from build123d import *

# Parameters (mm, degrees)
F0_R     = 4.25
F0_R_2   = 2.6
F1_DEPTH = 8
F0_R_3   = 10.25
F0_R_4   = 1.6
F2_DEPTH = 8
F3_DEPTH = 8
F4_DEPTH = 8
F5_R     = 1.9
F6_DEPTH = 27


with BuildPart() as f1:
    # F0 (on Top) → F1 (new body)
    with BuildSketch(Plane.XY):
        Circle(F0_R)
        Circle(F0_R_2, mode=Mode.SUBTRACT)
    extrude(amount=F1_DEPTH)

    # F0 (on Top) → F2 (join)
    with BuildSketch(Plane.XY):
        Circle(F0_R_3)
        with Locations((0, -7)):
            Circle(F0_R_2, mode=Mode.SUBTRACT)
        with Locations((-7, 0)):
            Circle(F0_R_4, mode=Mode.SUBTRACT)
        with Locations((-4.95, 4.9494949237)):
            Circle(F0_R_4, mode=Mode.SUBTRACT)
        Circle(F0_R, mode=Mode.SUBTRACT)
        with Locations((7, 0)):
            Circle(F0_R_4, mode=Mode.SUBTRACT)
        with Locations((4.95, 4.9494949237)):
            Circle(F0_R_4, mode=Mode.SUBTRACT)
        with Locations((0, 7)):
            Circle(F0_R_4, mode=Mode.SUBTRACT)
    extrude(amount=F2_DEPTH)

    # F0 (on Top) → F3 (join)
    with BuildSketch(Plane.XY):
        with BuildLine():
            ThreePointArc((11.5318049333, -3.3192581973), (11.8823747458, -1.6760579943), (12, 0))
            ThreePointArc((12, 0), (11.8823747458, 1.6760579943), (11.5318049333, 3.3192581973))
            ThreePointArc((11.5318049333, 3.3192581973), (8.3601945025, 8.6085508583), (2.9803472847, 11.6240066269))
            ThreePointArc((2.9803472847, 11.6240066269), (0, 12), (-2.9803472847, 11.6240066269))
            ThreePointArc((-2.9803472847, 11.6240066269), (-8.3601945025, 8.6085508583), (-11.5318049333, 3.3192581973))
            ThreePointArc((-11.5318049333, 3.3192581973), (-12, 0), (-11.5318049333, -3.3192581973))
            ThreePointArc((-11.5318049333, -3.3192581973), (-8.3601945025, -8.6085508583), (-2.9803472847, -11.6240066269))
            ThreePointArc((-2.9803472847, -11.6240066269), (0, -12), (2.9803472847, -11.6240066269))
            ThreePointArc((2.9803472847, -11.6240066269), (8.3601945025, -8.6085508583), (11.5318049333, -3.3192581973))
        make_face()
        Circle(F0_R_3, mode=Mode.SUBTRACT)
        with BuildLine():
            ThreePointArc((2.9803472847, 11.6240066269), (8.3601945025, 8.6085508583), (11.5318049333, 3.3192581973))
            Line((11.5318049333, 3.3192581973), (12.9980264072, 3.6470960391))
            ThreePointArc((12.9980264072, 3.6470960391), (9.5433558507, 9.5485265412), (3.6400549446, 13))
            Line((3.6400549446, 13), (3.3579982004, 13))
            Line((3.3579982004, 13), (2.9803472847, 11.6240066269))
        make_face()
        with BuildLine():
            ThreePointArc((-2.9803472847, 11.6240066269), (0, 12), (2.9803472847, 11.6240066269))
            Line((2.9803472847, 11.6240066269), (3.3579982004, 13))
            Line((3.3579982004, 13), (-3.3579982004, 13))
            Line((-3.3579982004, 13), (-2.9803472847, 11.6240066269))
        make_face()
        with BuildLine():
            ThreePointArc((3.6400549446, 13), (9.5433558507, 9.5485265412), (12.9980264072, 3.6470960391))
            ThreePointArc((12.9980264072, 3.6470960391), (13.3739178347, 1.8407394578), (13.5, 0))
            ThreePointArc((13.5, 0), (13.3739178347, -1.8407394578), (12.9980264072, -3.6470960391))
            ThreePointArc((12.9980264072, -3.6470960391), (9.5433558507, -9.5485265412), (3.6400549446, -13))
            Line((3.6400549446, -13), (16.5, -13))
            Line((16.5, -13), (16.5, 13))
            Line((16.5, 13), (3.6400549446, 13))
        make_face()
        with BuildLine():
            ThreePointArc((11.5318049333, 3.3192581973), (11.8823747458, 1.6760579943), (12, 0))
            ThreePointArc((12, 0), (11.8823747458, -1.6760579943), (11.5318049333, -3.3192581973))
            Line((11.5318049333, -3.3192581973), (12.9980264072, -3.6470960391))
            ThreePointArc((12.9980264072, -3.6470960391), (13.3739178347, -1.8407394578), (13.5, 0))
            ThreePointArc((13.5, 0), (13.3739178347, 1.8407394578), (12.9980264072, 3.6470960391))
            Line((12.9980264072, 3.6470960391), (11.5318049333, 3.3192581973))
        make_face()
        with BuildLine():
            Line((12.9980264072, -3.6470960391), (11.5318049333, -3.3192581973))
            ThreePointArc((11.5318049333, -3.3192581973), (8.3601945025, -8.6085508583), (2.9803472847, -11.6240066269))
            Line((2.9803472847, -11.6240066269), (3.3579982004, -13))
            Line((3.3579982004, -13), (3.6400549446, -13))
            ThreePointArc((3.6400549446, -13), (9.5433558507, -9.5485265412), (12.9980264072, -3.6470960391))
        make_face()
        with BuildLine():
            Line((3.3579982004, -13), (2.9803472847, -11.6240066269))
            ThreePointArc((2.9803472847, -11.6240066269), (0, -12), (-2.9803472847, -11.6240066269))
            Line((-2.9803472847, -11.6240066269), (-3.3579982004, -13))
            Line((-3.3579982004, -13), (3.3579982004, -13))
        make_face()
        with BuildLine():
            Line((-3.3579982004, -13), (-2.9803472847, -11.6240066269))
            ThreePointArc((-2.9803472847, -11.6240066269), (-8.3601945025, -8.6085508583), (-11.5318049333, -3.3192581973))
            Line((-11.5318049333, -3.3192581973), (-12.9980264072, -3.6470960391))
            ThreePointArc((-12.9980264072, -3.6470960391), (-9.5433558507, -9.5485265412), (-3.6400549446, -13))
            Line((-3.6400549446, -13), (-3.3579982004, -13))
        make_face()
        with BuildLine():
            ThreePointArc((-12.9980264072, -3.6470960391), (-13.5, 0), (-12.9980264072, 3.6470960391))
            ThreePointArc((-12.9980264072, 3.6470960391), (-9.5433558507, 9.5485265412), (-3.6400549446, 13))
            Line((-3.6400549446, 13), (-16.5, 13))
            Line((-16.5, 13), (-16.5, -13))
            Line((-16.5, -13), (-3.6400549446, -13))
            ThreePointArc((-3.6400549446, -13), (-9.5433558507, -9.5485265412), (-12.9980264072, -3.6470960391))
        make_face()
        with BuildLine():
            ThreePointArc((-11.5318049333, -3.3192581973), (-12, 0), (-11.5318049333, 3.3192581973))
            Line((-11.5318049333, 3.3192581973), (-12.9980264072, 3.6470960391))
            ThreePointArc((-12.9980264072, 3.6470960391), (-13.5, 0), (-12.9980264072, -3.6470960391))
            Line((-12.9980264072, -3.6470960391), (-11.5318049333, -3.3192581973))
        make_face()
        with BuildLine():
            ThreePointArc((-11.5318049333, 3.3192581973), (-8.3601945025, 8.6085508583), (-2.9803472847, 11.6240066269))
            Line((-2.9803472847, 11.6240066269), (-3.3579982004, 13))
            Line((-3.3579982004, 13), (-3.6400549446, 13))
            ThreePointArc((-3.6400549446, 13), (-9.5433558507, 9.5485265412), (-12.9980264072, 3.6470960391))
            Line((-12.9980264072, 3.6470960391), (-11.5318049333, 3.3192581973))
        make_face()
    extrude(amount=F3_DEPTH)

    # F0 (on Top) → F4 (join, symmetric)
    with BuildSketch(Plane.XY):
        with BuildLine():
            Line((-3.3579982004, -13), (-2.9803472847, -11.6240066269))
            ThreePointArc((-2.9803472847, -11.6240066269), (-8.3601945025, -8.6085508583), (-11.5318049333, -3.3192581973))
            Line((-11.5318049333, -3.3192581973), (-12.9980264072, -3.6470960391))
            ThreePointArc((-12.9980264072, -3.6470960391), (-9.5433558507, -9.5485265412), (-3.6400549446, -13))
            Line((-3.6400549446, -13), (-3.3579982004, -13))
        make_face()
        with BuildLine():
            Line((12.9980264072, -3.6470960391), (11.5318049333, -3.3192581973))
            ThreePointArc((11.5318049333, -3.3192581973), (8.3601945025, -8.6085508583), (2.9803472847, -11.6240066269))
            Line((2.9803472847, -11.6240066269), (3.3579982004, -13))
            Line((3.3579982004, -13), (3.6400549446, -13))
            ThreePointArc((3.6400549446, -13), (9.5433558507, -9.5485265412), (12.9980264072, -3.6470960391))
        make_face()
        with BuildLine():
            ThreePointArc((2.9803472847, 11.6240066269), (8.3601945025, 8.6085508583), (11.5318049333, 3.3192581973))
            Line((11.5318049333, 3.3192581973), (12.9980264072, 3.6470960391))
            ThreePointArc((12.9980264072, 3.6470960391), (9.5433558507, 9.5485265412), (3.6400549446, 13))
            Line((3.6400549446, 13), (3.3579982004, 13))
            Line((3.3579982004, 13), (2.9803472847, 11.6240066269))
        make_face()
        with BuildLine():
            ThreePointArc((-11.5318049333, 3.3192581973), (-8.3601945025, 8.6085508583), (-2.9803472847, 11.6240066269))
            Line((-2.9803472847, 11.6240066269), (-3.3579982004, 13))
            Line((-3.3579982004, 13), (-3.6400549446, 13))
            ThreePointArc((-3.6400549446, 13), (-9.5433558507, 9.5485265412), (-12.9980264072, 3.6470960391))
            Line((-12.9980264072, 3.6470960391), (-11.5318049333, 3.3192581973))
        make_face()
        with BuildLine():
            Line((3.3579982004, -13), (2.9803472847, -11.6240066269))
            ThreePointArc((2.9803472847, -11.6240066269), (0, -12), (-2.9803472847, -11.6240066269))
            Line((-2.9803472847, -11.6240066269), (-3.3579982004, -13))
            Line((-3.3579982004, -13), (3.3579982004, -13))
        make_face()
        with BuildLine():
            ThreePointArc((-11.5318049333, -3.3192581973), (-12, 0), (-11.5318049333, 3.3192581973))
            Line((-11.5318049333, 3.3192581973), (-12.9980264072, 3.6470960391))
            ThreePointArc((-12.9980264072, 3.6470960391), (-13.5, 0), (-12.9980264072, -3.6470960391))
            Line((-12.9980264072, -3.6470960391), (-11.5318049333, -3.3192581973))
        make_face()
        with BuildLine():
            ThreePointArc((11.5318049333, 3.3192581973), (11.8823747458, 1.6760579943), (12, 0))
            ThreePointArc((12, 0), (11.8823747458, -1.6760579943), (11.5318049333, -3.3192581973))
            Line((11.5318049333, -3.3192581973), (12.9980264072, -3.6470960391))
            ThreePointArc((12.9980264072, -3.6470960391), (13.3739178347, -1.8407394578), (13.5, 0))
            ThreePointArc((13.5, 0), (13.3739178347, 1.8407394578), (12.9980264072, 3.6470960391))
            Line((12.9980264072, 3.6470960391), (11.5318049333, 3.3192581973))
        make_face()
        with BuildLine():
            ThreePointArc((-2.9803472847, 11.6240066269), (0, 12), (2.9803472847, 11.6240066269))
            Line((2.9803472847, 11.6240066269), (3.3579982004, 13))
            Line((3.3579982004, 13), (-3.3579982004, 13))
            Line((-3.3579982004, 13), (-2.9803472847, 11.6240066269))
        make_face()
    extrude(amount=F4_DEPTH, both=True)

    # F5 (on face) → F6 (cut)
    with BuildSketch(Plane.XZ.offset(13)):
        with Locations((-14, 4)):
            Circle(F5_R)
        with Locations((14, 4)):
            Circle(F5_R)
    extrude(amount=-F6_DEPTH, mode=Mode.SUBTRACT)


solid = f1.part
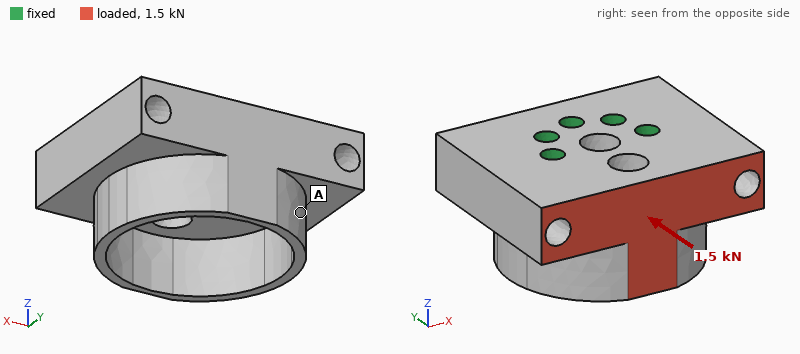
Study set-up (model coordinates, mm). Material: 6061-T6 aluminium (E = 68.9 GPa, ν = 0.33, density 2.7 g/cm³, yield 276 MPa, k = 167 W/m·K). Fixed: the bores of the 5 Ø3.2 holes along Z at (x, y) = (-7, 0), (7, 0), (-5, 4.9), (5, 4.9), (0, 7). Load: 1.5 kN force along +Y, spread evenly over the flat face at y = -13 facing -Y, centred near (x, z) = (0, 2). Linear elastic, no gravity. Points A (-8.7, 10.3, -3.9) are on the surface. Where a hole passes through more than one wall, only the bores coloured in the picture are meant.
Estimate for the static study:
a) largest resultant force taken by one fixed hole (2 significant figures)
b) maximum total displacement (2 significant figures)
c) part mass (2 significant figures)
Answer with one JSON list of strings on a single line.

["650 N", "35 µm", "18 g"]
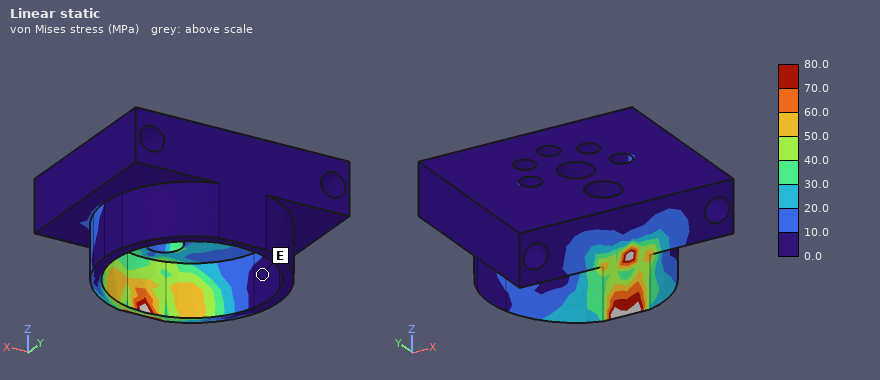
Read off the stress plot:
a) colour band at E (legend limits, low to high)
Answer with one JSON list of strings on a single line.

["0.0 to 10.0 MPa"]
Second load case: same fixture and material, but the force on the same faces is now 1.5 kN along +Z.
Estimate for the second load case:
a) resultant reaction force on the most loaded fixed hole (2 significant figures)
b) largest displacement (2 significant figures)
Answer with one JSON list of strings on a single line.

["960 N", "37 µm"]
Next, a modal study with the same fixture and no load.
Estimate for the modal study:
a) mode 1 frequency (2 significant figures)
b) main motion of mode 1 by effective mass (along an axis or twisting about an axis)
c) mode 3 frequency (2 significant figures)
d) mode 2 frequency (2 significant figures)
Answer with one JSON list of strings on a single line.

["24 kHz", "along Z", "30 kHz", "25 kHz"]
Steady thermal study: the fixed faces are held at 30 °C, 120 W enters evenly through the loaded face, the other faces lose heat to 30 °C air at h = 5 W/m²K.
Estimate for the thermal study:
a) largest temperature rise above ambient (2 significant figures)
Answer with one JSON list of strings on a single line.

["70 K"]
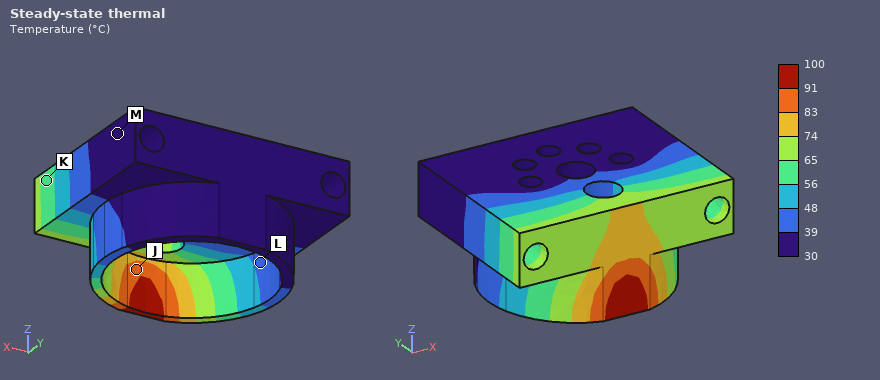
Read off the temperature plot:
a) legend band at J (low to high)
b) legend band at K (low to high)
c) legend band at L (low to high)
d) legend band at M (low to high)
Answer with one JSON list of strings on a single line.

["83 to 91 °C", "56 to 65 °C", "39 to 48 °C", "30 to 39 °C"]
